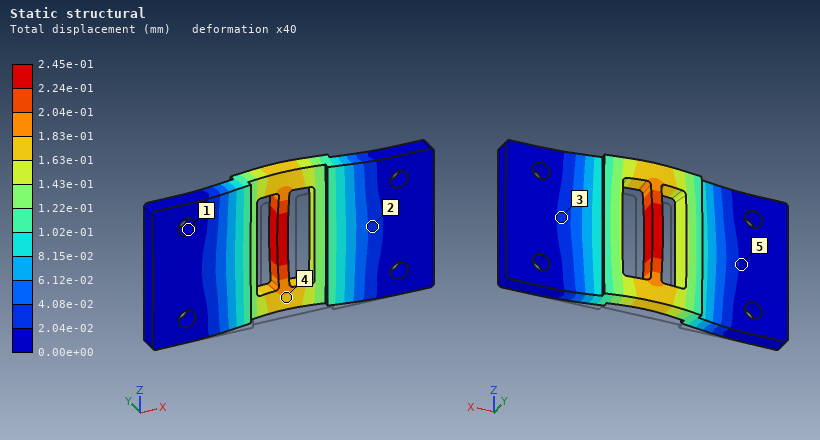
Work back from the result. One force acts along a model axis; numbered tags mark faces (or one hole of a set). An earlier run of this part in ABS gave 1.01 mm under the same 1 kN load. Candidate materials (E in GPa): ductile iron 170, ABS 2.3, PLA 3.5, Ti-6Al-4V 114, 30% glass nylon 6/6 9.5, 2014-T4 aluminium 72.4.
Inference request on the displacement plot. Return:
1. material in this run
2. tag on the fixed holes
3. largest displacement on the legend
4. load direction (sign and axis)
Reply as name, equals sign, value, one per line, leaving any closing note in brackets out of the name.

material in this run = 30% glass nylon 6/6
tag on the fixed holes = 1
largest displacement on the legend = 2.45e-01 mm
load direction = +Y
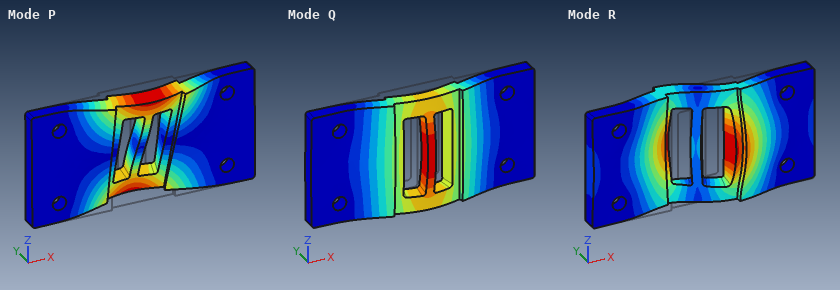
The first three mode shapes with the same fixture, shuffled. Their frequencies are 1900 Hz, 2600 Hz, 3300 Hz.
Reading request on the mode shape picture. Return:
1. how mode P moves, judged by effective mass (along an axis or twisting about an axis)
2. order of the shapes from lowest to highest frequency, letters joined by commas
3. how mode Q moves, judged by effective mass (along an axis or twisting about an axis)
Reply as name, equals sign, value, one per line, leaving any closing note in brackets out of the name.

how mode P moves, judged by effective mass = twisting about X
order of the shapes from lowest to highest frequency, letters joined by commas = Q, P, R
how mode Q moves, judged by effective mass = along Y
